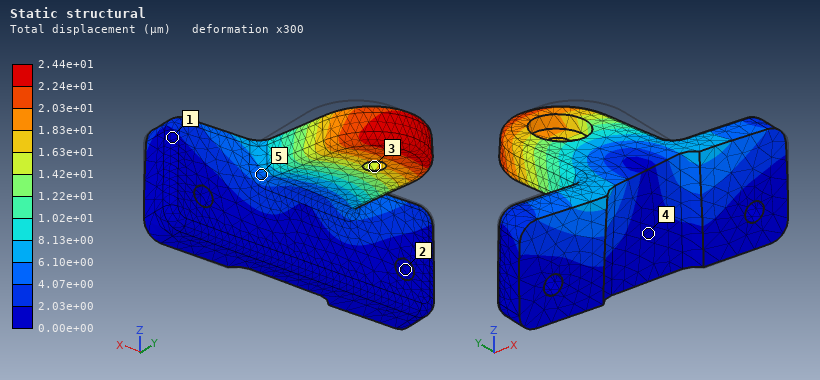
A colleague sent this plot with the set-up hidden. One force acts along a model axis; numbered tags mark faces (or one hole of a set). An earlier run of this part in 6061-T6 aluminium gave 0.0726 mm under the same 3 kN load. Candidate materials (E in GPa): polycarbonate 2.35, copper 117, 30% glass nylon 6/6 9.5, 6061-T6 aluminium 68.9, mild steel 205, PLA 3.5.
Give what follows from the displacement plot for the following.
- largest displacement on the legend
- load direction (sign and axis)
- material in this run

2.44e+01 µm
-X
mild steel
